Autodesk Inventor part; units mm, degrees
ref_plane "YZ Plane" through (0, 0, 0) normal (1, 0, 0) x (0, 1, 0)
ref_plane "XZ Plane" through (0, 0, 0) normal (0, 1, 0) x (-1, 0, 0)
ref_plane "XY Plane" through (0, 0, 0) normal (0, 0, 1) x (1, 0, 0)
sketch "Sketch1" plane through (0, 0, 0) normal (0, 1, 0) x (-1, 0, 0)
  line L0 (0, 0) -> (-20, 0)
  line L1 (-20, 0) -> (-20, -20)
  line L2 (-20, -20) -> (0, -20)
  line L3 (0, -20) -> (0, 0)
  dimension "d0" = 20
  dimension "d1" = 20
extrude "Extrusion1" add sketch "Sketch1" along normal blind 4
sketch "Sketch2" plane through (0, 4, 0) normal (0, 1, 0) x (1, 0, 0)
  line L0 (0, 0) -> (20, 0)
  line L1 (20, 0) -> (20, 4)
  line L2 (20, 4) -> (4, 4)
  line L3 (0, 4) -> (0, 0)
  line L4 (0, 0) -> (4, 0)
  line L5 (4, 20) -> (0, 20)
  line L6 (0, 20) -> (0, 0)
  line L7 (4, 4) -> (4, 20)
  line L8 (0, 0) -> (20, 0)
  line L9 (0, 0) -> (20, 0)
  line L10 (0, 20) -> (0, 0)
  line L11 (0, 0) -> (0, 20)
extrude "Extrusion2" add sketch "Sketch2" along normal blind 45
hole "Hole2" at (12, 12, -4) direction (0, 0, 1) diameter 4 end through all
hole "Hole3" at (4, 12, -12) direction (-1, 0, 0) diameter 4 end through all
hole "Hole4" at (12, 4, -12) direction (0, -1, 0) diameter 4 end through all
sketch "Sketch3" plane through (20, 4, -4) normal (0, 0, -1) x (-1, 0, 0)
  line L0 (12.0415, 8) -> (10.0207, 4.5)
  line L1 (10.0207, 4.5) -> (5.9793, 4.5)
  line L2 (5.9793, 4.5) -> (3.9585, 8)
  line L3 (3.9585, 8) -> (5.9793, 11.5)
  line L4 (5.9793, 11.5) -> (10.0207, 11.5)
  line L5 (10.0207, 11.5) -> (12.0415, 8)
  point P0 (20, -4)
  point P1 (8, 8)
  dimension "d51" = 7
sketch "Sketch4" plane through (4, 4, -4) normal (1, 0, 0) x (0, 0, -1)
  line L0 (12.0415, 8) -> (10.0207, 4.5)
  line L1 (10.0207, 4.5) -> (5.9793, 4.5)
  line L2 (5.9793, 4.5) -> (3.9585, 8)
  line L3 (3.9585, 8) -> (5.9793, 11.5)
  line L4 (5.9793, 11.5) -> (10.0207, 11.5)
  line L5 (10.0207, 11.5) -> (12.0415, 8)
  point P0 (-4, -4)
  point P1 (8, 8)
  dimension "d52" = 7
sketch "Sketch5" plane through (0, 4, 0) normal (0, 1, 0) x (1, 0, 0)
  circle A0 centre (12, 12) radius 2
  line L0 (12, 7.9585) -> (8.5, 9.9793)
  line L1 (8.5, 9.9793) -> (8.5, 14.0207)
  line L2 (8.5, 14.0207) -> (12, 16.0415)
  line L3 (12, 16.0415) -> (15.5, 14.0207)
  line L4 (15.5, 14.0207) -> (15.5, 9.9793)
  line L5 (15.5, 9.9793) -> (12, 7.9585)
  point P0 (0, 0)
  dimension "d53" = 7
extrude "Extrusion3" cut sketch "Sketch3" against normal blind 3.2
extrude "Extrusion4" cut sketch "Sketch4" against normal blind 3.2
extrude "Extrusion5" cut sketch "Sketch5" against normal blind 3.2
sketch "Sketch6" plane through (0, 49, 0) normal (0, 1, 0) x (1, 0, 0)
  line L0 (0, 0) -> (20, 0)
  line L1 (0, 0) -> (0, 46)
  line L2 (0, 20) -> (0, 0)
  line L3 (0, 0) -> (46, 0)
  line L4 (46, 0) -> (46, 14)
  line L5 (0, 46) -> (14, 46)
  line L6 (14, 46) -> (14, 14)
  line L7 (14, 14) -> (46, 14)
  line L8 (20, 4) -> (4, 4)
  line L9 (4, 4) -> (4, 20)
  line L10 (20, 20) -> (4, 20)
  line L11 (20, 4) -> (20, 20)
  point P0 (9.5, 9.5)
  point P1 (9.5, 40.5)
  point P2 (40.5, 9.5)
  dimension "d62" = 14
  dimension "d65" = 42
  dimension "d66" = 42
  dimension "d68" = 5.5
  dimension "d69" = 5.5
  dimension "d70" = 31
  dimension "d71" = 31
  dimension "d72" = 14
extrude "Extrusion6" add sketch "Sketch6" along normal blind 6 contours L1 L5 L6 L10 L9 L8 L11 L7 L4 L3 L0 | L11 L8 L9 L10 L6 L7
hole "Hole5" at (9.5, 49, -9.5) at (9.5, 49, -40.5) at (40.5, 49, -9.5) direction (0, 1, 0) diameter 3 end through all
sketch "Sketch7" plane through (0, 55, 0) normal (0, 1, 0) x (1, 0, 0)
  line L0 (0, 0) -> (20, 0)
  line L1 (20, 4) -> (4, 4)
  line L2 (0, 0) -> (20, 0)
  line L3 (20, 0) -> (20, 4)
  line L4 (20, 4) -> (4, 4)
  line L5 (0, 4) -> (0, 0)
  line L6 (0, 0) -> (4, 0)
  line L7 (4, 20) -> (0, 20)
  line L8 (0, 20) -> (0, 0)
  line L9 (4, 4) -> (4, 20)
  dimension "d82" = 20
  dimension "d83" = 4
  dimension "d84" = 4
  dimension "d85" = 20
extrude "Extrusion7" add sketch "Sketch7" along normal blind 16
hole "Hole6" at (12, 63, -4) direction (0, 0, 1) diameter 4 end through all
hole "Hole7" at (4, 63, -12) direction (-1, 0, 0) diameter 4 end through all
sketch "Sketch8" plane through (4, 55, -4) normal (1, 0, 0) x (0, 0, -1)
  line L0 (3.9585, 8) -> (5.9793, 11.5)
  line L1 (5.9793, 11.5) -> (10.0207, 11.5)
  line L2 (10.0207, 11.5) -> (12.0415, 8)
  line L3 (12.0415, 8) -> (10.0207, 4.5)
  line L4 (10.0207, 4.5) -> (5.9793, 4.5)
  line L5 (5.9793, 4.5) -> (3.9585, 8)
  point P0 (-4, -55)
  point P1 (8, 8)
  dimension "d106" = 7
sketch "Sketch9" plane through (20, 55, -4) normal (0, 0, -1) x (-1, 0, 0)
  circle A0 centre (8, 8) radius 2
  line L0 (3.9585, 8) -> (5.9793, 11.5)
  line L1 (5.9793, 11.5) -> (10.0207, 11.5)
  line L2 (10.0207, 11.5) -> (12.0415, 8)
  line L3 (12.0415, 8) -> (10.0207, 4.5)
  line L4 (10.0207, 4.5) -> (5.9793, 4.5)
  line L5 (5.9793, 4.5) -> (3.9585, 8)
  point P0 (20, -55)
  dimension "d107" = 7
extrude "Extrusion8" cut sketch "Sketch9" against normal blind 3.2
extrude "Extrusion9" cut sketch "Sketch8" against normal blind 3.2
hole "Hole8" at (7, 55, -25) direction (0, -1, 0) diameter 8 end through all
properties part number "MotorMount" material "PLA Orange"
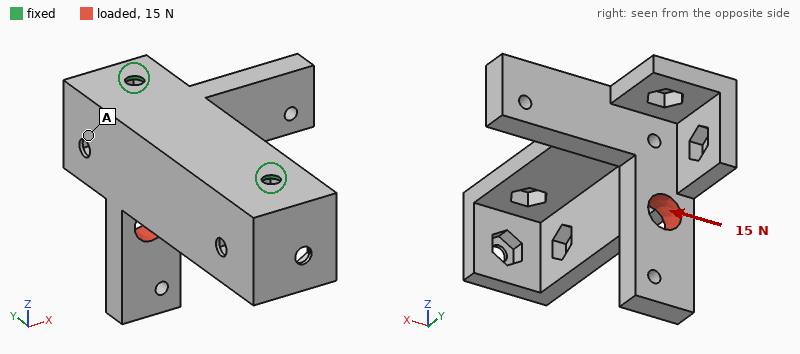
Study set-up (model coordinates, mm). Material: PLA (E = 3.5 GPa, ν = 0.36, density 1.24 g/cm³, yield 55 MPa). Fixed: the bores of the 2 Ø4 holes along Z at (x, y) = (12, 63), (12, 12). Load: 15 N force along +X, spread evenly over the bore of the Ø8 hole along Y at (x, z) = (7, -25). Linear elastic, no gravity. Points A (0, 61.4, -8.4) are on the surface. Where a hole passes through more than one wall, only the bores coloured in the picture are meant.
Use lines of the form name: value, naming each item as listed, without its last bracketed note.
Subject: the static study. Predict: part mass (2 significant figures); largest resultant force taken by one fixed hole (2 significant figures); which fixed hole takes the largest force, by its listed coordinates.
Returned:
part mass: 20 g
largest resultant force taken by one fixed hole: 14 N
which fixed hole takes the largest force, by its listed coordinates: (12, 63)
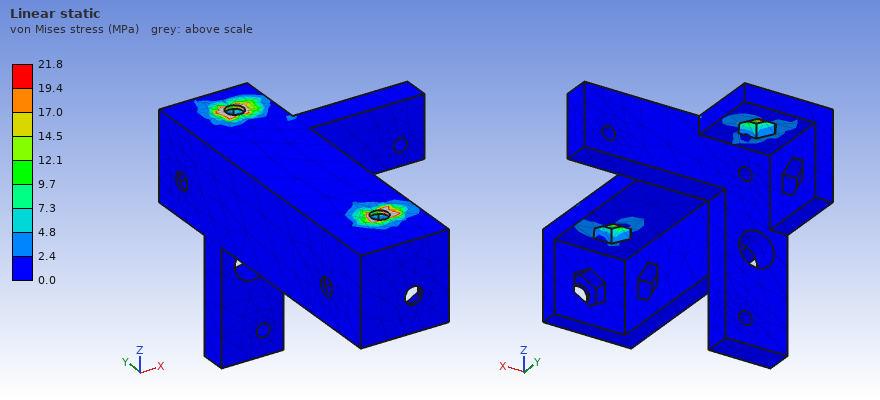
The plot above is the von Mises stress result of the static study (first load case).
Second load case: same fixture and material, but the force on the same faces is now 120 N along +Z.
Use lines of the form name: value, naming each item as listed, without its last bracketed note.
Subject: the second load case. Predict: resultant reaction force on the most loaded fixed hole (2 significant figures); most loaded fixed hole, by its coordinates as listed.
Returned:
resultant reaction force on the most loaded fixed hole: 99 N
most loaded fixed hole, by its coordinates as listed: (12, 63)
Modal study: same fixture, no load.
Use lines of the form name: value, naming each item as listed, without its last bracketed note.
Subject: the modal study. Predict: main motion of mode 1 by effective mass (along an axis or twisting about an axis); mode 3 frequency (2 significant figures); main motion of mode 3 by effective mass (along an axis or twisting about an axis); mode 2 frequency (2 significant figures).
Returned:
main motion of mode 1 by effective mass: along X
mode 3 frequency: 1400 Hz
main motion of mode 3 by effective mass: along Z
mode 2 frequency: 970 Hz
